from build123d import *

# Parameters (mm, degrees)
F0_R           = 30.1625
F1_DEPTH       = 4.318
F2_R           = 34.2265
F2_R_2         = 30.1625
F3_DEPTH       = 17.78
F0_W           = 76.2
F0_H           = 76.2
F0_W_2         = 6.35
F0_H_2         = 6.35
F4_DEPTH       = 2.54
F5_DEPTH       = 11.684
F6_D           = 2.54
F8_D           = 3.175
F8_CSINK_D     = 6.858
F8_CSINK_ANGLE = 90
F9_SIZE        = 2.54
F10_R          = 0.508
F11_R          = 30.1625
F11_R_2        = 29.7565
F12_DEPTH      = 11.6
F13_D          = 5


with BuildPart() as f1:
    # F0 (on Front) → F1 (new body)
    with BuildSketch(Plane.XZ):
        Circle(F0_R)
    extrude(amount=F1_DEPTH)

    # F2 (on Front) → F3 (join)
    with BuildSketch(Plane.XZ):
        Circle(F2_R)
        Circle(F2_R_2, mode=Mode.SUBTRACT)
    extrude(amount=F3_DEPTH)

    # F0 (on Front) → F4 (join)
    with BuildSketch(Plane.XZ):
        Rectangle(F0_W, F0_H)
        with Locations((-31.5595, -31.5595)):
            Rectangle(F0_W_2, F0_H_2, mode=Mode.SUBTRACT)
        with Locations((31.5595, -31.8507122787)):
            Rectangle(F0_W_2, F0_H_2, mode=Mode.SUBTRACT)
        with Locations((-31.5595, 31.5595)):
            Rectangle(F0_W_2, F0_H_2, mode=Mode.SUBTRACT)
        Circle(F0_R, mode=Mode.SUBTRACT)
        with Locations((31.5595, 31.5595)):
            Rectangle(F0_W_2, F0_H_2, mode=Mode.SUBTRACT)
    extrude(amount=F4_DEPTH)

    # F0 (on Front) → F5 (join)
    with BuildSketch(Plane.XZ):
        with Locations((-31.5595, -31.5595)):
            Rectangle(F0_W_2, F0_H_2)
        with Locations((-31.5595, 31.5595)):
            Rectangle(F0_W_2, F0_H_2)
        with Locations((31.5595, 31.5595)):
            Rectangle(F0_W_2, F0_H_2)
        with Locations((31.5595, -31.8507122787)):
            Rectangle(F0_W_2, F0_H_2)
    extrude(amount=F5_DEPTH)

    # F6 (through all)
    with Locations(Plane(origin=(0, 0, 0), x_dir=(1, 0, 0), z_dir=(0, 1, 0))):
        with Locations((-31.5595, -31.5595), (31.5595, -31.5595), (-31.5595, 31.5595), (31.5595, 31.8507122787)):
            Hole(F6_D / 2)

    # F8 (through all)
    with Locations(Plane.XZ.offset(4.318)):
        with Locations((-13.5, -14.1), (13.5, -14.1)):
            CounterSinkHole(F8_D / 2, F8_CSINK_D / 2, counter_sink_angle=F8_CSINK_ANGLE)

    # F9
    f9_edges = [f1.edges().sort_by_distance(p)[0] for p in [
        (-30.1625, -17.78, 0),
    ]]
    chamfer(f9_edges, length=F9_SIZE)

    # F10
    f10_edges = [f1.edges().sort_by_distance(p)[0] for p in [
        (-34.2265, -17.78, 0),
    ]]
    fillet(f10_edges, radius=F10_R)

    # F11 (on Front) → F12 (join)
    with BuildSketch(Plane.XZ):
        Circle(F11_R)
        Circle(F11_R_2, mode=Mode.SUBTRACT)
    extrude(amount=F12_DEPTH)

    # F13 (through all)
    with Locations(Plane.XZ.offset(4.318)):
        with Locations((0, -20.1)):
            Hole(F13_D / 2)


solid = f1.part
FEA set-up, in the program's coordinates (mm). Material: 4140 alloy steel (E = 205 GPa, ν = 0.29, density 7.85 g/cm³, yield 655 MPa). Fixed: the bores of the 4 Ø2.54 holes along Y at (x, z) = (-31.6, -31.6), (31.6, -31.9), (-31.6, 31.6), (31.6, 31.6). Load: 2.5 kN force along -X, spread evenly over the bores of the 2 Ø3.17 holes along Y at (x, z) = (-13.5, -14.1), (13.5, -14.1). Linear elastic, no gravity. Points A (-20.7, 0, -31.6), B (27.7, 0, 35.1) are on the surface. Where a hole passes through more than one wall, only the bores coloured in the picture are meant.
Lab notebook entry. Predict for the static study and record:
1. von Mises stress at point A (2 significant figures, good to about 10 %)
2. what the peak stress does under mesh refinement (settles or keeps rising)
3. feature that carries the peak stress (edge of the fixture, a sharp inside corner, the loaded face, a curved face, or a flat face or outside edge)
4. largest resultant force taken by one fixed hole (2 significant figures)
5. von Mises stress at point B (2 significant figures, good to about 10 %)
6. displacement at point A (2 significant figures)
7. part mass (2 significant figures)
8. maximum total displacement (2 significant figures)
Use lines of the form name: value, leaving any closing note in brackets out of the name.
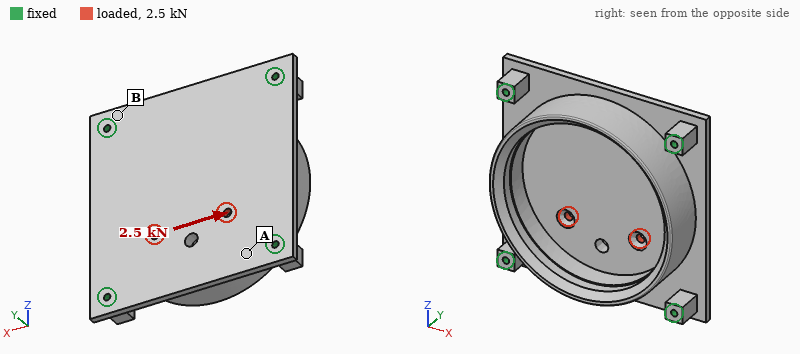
von Mises stress at point A: 17 MPa
what the peak stress does under mesh refinement: keeps rising
feature that carries the peak stress: edge of the fixture
largest resultant force taken by one fixed hole: 860 N
von Mises stress at point B: 6.9 MPa
displacement at point A: 1.2 µm
part mass: 260 g
maximum total displacement: 3.6 µm
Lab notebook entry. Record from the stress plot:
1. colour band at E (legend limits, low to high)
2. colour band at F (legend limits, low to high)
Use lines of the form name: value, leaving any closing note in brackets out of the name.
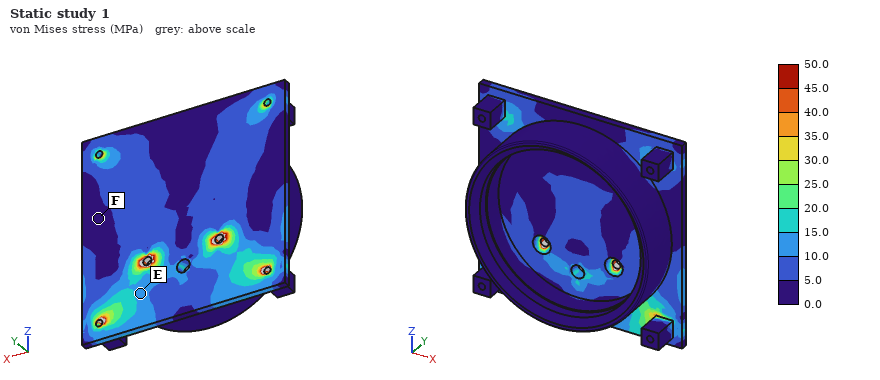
colour band at E: 10.0 to 15.0 MPa
colour band at F: 0.0 to 5.0 MPa
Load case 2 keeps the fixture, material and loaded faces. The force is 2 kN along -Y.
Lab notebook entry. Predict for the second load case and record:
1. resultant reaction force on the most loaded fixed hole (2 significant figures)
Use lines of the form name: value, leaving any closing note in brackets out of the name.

resultant reaction force on the most loaded fixed hole: 830 N
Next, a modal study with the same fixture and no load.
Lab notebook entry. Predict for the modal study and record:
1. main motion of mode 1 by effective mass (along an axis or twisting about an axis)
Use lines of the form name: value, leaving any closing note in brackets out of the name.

main motion of mode 1 by effective mass: along Y
